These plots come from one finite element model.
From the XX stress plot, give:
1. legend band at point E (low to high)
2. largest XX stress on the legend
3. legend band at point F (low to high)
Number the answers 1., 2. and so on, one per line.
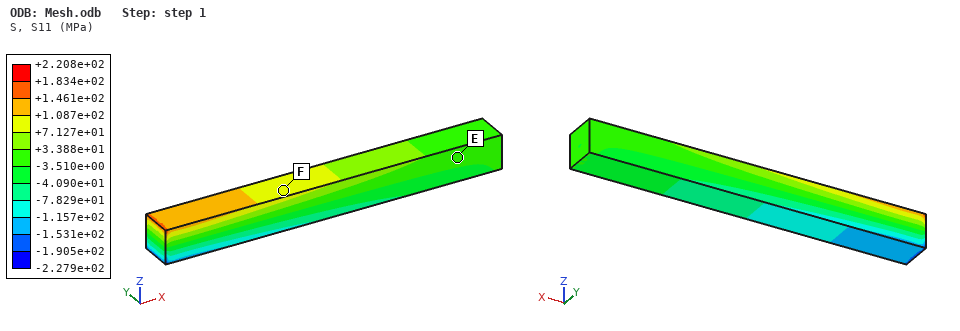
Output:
1. -3.510e+00 to +3.388e+01 MPa
2. +2.208e+02 MPa
3. +7.127e+01 to +1.087e+02 MPa
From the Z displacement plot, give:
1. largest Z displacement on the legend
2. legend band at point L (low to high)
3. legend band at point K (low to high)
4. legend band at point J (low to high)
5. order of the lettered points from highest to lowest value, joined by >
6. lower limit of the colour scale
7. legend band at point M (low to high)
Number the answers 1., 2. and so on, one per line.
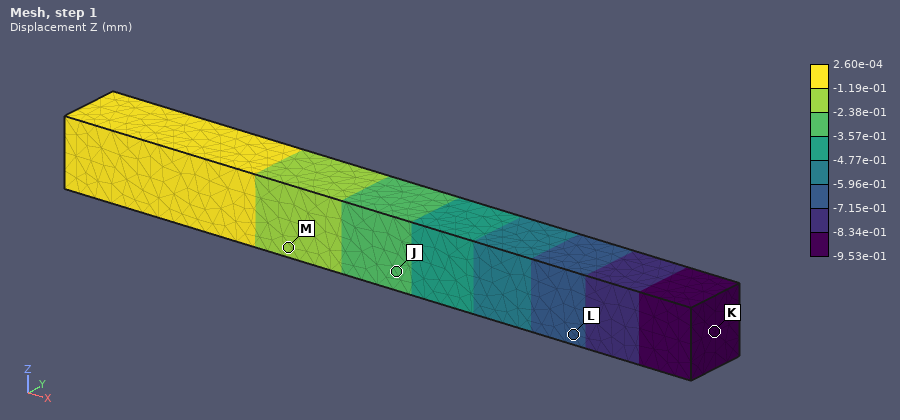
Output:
1. 2.60e-04 mm
2. -7.15e-01 to -5.96e-01 mm
3. -9.53e-01 to -8.34e-01 mm
4. -3.57e-01 to -2.38e-01 mm
5. M > J > L > K
6. -9.53e-01 mm
7. -2.38e-01 to -1.19e-01 mm
